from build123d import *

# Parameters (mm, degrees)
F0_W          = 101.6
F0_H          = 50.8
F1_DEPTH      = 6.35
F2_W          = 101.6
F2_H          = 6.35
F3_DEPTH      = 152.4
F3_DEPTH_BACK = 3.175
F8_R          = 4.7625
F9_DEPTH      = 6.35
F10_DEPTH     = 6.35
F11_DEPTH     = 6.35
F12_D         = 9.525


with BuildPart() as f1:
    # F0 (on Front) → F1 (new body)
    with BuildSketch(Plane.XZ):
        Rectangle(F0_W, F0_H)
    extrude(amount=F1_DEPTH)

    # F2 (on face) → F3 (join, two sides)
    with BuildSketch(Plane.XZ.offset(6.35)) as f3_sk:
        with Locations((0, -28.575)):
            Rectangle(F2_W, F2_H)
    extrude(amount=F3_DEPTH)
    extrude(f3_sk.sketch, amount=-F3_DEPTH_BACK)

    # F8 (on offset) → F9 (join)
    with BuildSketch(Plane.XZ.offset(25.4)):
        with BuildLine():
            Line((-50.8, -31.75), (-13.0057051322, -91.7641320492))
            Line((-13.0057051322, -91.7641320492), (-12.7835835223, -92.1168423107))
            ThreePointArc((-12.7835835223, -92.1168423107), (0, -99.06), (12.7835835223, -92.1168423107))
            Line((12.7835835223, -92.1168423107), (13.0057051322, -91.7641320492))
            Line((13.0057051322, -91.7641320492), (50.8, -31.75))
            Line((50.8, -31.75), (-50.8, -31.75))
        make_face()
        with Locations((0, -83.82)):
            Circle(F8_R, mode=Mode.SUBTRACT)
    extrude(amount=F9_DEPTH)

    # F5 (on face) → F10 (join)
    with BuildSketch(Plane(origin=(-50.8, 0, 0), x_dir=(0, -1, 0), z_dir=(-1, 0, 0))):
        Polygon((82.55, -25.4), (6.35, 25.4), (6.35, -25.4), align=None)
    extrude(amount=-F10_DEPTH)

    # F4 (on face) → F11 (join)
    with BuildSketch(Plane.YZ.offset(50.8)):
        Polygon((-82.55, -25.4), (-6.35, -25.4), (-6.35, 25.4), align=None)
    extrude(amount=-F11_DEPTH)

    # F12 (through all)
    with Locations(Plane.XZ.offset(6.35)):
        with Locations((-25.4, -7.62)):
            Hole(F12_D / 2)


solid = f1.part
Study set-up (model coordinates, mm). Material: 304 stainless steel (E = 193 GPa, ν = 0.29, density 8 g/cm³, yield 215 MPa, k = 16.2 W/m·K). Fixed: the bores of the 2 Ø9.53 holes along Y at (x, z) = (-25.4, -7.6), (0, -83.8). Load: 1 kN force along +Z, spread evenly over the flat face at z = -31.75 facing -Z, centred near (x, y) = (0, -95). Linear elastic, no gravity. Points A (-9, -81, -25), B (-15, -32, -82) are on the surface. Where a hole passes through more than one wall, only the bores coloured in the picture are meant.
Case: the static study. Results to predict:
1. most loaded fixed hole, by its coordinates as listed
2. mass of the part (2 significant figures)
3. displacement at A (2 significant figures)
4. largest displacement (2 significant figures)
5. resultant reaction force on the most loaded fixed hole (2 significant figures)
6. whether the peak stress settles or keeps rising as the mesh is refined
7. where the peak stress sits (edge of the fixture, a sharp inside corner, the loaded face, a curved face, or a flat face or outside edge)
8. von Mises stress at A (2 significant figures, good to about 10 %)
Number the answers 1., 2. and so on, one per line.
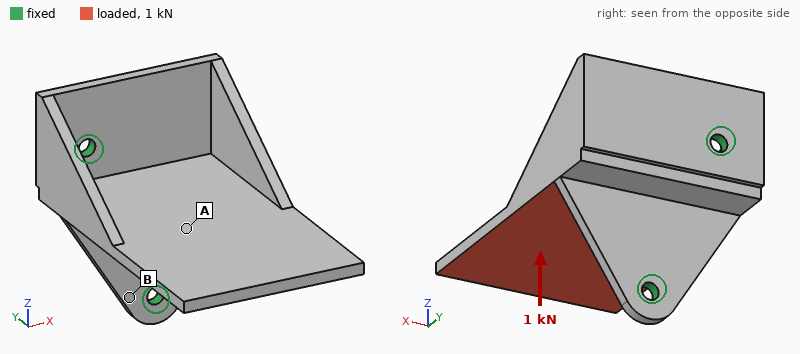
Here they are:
1. (0, -83.8)
2. 1.5 kg
3. 0.072 mm
4. 0.32 mm
5. 2.7 kN
6. keeps rising
7. edge of the fixture
8. 23 MPa
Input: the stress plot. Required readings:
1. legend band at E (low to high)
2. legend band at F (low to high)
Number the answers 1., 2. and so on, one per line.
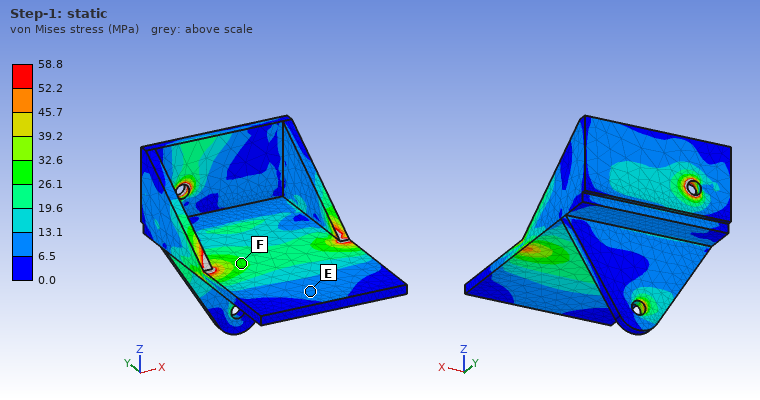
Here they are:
1. 6.5 to 13.1 MPa
2. 26.1 to 32.6 MPa
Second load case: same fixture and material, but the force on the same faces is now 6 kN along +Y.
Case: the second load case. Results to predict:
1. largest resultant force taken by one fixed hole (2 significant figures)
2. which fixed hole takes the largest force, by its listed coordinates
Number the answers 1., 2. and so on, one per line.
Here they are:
1. 6.2 kN
2. (-25.4, -7.6)
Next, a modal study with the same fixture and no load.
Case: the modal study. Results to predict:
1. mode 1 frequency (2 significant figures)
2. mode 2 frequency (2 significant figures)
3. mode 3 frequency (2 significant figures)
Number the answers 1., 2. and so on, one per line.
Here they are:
1. 410 Hz
2. 500 Hz
3. 1100 Hz
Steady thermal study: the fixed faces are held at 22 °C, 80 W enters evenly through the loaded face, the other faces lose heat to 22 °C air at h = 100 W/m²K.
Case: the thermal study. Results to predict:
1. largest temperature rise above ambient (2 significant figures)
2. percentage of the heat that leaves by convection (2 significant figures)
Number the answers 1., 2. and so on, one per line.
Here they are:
1. 54 K
2. 98 %
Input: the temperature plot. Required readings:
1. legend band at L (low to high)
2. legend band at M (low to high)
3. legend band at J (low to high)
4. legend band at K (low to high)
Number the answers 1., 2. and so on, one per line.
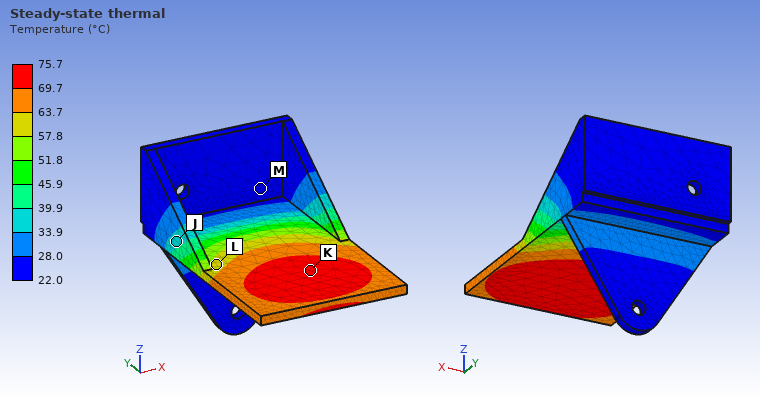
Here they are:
1. 57.8 to 63.7 °C
2. 22.0 to 28.0 °C
3. 33.9 to 39.9 °C
4. 69.7 to 75.7 °C
